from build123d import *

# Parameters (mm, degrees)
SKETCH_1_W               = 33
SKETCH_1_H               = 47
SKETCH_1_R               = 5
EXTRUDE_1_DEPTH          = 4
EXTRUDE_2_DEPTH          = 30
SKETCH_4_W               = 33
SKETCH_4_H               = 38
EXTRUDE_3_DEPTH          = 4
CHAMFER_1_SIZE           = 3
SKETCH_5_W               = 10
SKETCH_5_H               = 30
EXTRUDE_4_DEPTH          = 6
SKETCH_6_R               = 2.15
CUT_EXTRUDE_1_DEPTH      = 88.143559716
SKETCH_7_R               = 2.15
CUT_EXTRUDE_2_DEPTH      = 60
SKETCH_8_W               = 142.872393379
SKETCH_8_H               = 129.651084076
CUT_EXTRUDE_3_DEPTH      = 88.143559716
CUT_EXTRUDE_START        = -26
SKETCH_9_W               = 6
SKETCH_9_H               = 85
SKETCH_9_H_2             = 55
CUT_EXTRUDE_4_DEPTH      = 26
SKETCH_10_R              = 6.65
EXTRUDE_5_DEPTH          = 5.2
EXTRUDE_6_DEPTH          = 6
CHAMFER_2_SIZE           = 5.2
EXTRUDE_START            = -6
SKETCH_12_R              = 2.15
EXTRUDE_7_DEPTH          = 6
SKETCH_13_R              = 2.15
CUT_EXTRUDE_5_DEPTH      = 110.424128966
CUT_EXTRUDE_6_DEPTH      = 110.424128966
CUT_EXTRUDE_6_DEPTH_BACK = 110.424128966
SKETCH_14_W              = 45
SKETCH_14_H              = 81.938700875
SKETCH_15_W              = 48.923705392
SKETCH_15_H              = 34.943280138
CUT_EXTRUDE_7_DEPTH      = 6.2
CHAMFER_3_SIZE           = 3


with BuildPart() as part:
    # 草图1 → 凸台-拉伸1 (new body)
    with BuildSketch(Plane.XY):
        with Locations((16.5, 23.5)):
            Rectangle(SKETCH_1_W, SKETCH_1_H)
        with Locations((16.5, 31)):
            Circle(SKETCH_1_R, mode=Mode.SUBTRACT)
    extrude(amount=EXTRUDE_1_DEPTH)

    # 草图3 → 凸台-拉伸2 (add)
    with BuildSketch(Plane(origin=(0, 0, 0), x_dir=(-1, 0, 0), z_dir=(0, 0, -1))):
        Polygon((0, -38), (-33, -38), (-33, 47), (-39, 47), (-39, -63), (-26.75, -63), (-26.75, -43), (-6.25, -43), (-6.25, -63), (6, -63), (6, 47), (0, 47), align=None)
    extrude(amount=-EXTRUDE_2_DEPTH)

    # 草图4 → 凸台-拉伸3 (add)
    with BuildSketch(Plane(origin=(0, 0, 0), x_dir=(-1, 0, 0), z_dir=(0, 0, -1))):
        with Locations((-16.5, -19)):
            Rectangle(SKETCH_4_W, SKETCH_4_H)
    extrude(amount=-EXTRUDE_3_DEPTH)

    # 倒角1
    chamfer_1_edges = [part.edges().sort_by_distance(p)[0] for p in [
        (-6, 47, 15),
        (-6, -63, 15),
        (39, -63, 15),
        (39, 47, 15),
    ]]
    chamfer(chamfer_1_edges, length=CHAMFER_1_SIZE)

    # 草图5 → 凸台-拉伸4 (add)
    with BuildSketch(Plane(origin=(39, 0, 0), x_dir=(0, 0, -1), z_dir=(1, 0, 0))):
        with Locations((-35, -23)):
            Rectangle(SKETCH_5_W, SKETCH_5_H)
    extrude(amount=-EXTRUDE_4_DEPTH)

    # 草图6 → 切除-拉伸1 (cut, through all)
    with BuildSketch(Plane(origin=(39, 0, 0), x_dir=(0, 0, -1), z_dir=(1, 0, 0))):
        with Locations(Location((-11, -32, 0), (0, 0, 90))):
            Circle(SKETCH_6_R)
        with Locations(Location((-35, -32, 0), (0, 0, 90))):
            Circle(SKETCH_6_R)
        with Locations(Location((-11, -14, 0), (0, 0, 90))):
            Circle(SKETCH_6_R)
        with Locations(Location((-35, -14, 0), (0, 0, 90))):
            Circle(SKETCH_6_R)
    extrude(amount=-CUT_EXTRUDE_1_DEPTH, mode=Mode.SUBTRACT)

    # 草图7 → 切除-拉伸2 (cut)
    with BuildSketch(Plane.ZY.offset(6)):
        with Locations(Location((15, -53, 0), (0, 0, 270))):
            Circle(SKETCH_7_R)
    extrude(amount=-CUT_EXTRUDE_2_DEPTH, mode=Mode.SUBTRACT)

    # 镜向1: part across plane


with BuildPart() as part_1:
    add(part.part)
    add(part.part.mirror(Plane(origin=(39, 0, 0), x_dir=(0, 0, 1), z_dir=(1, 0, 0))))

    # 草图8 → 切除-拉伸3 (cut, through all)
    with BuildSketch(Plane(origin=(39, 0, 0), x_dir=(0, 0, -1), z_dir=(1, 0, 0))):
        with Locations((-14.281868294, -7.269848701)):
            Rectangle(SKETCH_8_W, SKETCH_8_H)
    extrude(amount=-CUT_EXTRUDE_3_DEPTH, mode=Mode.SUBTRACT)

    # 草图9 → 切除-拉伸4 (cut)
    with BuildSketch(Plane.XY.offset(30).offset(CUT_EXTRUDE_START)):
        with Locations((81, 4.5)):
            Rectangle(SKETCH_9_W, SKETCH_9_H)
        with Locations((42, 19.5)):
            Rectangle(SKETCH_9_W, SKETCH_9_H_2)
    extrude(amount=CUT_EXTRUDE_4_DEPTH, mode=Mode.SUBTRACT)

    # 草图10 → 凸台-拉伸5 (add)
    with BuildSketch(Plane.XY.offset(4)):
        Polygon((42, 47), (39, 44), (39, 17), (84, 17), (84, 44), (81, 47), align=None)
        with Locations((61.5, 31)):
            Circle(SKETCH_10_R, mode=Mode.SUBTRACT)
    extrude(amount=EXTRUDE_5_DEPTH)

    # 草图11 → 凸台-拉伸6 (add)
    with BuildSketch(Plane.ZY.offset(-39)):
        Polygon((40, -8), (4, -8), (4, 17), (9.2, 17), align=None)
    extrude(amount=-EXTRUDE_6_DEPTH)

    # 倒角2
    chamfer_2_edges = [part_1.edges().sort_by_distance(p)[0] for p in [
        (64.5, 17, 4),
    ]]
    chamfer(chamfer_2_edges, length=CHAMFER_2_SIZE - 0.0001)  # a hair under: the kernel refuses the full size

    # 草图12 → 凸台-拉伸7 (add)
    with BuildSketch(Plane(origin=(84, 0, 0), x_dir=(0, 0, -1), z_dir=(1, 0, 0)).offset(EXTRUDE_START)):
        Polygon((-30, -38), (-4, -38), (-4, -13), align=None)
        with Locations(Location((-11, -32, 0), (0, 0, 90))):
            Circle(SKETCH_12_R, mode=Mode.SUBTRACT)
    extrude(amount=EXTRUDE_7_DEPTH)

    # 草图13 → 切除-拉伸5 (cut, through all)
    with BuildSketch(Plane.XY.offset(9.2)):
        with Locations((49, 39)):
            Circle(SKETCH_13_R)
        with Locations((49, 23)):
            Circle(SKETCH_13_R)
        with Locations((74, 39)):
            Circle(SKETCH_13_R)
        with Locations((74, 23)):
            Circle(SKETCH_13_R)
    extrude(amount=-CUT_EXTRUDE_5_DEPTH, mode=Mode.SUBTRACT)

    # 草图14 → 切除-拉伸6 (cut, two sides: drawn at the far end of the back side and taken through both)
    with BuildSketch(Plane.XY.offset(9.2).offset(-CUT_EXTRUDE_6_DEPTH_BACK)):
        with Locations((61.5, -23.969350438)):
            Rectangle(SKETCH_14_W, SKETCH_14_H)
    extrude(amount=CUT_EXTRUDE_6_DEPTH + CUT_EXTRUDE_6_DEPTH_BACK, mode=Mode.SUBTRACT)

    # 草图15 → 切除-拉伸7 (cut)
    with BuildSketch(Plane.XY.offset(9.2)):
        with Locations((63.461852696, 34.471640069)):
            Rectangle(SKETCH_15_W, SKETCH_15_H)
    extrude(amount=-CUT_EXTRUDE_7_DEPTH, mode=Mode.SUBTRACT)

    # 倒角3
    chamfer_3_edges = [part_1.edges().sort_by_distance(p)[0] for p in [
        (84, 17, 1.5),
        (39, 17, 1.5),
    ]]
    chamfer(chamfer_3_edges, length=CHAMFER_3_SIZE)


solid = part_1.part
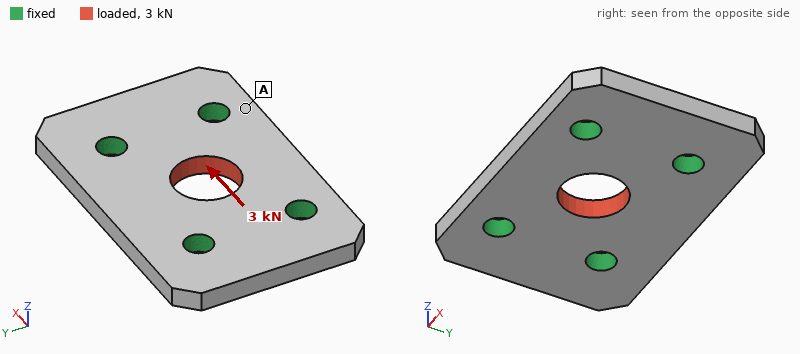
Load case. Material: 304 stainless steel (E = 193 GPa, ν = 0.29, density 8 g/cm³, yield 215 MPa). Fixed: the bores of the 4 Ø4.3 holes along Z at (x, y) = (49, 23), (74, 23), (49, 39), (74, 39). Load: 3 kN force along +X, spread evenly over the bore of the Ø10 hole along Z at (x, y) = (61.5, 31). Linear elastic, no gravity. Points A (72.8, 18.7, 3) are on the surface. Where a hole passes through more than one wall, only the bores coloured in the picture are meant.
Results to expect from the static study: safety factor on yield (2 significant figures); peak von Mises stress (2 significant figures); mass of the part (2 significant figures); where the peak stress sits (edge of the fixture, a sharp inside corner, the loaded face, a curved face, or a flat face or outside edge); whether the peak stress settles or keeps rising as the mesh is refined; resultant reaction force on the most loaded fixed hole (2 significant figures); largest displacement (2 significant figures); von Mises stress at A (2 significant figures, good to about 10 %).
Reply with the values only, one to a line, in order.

3.9
55 MPa
29 g
the loaded face
settles
790 N
1.6 µm
6.4 MPa
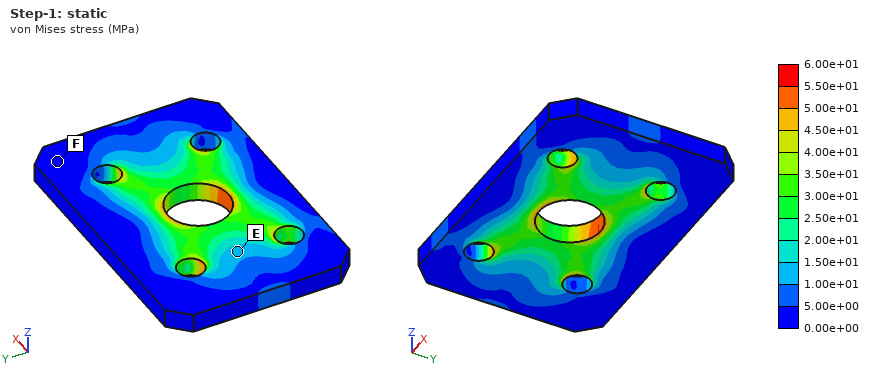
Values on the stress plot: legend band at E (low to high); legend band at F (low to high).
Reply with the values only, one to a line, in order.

1.00e+01 to 1.50e+01 MPa
0.00e+00 to 5.00e+00 MPa
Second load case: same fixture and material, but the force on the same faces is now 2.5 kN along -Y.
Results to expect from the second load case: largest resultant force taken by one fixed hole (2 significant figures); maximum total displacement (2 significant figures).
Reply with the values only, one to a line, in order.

700 N
2.6 µm
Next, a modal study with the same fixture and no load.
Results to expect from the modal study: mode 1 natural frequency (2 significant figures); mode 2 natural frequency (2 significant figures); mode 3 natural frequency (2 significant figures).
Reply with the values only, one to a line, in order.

24 kHz
26 kHz
27 kHz
